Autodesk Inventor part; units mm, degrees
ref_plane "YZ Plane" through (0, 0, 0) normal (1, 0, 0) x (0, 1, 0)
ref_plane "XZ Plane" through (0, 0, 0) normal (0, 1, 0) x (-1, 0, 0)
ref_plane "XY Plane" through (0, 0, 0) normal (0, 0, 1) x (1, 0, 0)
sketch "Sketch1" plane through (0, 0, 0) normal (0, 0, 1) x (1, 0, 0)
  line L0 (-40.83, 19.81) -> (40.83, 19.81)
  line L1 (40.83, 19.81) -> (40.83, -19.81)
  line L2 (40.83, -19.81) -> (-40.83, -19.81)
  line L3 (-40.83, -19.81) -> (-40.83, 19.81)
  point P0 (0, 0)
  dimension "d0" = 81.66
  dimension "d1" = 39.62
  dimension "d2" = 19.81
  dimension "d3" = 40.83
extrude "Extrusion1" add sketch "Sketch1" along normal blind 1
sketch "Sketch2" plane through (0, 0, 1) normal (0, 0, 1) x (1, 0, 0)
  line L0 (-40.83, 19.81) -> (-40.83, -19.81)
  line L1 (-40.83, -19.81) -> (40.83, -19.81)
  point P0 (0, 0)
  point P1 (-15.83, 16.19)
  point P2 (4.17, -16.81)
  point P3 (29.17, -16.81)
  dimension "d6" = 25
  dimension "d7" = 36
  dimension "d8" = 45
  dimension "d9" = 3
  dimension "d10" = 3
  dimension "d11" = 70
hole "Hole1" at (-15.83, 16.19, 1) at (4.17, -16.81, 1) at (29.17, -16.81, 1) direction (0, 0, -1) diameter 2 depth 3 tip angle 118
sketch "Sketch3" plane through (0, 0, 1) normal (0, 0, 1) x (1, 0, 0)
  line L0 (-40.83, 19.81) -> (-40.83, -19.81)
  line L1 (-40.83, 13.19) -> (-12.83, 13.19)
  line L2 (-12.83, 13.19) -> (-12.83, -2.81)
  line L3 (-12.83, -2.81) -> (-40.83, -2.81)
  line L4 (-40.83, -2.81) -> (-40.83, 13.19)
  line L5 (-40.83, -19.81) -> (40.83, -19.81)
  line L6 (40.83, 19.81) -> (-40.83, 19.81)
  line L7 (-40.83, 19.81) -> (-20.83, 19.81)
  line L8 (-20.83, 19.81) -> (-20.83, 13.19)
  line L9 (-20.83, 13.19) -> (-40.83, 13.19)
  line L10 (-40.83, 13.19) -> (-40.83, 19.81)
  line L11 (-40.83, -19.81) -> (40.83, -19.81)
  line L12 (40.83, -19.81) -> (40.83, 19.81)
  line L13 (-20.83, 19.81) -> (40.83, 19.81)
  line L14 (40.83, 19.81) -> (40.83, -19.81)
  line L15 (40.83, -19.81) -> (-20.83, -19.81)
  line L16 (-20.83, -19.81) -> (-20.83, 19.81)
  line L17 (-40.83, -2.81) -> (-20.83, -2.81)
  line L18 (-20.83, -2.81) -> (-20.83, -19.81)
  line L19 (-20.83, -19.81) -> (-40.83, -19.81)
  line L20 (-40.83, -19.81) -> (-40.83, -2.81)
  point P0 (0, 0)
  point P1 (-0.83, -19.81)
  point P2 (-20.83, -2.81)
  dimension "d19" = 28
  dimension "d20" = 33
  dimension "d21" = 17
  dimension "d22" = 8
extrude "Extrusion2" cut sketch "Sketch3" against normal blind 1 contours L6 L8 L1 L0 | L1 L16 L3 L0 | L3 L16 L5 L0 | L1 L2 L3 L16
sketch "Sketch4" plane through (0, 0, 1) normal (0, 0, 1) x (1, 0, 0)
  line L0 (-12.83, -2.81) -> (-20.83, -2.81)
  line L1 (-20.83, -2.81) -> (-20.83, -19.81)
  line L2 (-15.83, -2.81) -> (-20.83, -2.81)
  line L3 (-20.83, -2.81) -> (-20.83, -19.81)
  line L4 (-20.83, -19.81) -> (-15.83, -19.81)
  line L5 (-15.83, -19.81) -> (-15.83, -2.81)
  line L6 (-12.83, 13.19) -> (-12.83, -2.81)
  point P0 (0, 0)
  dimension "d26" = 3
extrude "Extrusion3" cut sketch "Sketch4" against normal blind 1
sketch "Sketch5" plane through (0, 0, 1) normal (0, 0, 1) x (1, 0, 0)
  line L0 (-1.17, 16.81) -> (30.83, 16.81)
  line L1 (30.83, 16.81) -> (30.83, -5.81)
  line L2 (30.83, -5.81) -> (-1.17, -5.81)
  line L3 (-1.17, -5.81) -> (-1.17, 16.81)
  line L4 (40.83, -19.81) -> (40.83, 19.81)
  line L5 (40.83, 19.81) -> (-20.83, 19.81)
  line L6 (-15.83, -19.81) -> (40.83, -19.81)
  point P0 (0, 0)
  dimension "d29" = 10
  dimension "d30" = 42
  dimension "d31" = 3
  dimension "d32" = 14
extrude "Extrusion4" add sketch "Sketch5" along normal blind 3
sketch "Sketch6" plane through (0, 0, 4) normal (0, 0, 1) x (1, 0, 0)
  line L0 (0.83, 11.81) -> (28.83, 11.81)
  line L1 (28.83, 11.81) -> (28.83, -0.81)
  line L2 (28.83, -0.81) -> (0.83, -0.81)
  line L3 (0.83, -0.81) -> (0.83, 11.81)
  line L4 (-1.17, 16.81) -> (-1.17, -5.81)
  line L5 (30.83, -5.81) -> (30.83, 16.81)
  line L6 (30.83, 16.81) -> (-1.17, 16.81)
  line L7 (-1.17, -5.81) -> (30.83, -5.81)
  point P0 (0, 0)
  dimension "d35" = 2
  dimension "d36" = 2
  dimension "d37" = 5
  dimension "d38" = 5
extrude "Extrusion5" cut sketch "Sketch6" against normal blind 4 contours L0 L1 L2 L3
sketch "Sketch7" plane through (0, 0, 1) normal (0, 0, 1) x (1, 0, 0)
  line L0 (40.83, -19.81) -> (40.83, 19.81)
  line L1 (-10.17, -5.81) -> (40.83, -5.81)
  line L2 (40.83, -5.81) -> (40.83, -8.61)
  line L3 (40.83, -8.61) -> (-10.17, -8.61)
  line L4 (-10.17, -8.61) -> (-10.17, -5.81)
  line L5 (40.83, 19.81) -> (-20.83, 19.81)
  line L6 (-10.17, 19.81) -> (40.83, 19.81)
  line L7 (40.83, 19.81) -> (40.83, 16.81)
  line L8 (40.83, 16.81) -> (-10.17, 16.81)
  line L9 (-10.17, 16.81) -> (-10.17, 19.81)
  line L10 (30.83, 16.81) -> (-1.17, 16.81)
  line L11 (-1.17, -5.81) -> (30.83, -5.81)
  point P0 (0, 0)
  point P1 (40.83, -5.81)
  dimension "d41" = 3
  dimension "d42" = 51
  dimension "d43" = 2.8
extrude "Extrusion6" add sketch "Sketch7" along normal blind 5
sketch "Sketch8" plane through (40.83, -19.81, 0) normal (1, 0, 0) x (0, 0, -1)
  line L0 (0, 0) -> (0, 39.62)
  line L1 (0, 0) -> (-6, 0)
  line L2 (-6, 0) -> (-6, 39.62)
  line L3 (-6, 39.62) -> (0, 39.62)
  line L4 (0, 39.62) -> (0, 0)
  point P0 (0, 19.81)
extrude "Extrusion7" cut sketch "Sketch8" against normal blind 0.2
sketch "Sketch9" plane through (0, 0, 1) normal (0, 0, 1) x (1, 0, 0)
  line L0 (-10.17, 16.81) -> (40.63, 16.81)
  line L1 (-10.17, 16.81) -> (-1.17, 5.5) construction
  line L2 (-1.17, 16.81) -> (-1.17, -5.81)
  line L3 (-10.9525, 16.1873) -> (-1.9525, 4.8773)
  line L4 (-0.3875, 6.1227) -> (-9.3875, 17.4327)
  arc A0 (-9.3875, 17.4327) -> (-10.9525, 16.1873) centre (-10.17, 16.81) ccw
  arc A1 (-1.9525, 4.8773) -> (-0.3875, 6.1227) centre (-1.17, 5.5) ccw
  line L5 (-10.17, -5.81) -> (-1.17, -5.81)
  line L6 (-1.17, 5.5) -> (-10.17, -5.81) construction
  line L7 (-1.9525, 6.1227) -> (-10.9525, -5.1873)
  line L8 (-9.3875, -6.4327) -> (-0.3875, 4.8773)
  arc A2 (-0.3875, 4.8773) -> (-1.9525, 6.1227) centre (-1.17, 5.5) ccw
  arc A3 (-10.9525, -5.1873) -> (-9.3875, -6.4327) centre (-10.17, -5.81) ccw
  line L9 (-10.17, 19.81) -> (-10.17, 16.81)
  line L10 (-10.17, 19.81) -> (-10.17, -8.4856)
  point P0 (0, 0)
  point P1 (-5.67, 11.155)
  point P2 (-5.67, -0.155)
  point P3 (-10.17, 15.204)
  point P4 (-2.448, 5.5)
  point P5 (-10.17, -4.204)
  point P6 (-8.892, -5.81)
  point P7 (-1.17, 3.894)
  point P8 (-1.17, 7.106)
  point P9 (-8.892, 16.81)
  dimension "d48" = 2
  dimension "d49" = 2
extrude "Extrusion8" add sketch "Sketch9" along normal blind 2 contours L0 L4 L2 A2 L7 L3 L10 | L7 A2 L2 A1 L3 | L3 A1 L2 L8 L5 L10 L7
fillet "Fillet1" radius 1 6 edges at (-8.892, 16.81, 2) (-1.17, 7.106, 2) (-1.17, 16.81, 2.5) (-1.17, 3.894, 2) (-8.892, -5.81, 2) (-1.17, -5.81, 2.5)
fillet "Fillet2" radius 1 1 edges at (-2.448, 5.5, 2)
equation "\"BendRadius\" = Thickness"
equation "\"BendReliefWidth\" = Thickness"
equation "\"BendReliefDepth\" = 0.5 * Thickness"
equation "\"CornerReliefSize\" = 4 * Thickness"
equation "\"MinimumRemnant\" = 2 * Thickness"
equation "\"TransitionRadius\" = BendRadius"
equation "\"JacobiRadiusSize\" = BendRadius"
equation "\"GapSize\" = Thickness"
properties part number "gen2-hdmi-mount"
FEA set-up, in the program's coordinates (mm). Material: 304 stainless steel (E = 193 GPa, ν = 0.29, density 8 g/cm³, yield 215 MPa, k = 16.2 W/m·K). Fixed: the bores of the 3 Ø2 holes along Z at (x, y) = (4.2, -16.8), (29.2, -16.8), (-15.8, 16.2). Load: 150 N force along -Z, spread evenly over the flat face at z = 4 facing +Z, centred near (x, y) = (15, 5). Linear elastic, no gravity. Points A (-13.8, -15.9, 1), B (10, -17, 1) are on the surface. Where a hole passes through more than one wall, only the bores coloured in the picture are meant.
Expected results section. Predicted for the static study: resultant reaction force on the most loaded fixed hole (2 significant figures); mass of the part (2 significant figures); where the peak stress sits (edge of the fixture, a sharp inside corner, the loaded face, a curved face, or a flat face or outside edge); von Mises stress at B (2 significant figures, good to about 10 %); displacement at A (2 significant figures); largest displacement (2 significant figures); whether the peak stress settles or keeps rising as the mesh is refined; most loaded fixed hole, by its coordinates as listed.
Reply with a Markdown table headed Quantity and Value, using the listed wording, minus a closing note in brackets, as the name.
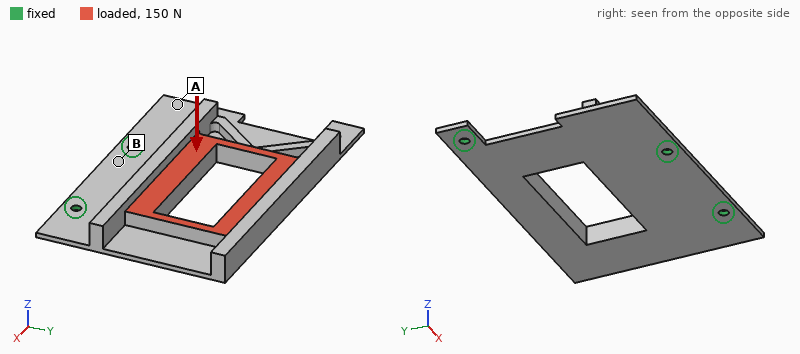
| Quantity | Value |
|---|---|
| resultant reaction force on the most loaded fixed hole | 190 N |
| mass of the part | 37 g |
| where the peak stress sits | edge of the fixture |
| von Mises stress at B | 39 MPa |
| displacement at A | 0.042 mm |
| largest displacement | 0.24 mm |
| whether the peak stress settles or keeps rising as the mesh is refined | keeps rising |
| most loaded fixed hole, by its coordinates as listed | (29.2, -16.8) |
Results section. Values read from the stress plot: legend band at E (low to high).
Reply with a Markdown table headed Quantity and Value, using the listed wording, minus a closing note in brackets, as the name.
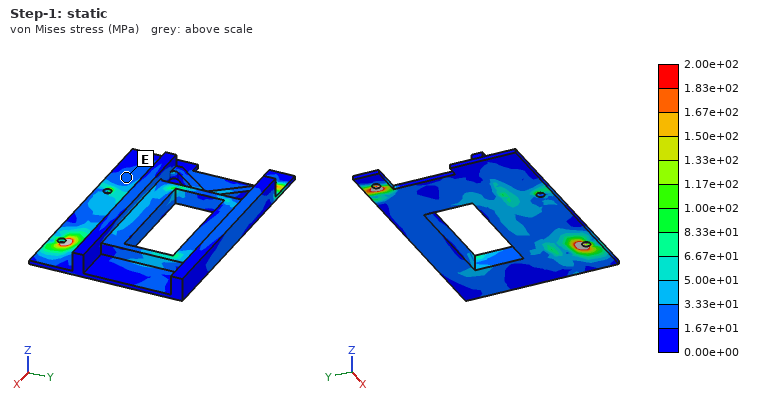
| Quantity | Value |
|---|---|
| legend band at E | 1.67e+01 to 3.33e+01 MPa |
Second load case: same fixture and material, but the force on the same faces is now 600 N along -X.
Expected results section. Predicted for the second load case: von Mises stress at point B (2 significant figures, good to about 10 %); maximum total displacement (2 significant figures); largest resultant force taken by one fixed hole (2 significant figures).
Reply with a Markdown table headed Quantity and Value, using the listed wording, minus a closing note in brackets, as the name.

| Quantity | Value |
|---|---|
| von Mises stress at point B | 29 MPa |
| maximum total displacement | 0.14 mm |
| largest resultant force taken by one fixed hole | 260 N |
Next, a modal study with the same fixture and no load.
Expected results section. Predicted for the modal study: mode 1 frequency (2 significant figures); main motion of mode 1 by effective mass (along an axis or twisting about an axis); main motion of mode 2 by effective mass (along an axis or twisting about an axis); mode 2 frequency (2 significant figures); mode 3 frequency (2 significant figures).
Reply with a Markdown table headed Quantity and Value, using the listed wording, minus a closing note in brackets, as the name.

| Quantity | Value |
|---|---|
| mode 1 frequency | 970 Hz |
| main motion of mode 1 by effective mass | along Z |
| main motion of mode 2 by effective mass | along Z |
| mode 2 frequency | 3400 Hz |
| mode 3 frequency | 4500 Hz |
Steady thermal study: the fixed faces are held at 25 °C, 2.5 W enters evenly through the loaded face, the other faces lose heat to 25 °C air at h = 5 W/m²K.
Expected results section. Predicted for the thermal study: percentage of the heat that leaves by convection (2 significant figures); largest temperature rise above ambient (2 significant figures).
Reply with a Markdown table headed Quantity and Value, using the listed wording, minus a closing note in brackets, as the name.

| Quantity | Value |
|---|---|
| percentage of the heat that leaves by convection | 28 % |
| largest temperature rise above ambient | 49 K |
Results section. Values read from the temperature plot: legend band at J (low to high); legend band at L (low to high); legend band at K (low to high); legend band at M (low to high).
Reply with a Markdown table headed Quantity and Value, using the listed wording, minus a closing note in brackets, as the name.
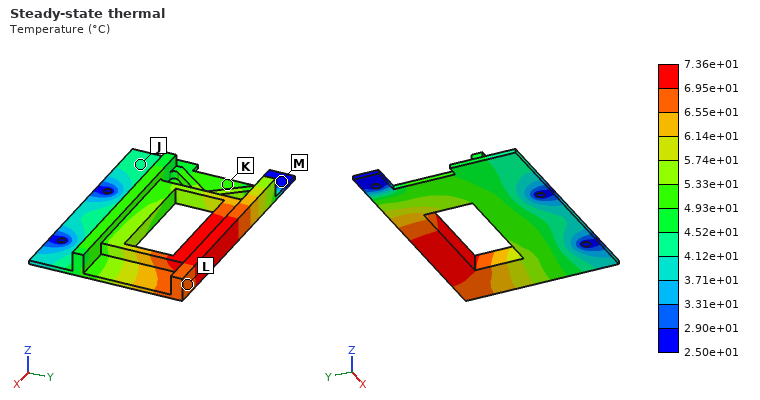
| Quantity | Value |
|---|---|
| legend band at J | 4.12e+01 to 4.52e+01 °C |
| legend band at L | 6.55e+01 to 6.95e+01 °C |
| legend band at K | 4.93e+01 to 5.33e+01 °C |
| legend band at M | 2.50e+01 to 2.90e+01 °C |
